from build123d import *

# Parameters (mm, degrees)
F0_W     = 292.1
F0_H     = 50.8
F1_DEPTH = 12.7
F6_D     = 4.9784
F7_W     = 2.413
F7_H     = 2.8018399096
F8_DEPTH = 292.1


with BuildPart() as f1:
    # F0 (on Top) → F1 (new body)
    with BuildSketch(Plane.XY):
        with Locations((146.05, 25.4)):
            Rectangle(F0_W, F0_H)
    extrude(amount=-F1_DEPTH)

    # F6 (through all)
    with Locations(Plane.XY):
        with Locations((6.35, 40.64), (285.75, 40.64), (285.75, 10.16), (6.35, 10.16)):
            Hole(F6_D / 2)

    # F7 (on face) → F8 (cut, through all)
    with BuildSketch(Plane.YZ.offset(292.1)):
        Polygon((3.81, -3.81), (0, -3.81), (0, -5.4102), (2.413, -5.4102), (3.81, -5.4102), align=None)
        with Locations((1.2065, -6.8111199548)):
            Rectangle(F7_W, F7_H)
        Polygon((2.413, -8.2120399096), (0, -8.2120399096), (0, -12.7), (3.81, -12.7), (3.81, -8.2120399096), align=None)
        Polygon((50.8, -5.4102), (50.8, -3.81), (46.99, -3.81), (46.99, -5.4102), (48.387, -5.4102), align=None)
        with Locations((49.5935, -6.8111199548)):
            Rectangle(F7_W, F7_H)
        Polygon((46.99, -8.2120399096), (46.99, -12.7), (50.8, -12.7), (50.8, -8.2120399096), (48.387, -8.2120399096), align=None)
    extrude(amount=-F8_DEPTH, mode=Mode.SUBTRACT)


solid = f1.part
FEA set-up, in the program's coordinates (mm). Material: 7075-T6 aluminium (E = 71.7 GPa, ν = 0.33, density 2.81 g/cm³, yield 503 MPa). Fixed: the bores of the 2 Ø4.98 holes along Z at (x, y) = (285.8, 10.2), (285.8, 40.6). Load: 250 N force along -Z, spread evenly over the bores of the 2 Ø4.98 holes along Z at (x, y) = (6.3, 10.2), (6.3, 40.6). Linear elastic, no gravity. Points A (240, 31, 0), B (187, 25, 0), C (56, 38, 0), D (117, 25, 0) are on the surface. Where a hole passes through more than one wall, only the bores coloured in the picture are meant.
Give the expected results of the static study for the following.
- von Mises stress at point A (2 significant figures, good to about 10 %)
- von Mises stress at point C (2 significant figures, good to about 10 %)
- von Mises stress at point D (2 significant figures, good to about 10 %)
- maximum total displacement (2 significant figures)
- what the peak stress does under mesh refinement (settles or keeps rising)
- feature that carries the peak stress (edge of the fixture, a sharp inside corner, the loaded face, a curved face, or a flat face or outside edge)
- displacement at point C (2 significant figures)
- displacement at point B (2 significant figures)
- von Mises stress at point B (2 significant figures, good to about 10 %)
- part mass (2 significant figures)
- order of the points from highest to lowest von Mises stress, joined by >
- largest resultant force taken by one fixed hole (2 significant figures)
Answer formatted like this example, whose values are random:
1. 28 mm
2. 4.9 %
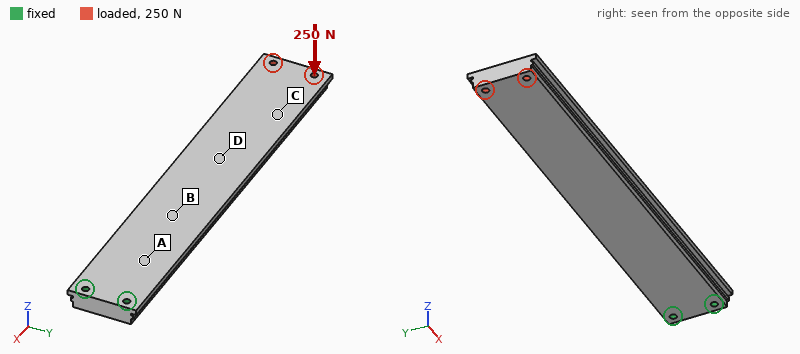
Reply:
1. 45 MPa
2. 9.6 MPa
3. 21 MPa
4. 3.4 mm
5. keeps rising
6. edge of the fixture
7. 2.4 mm
8. 0.57 mm
9. 35 MPa
10. 480 g
11. A > B > D > C
12. 210 N
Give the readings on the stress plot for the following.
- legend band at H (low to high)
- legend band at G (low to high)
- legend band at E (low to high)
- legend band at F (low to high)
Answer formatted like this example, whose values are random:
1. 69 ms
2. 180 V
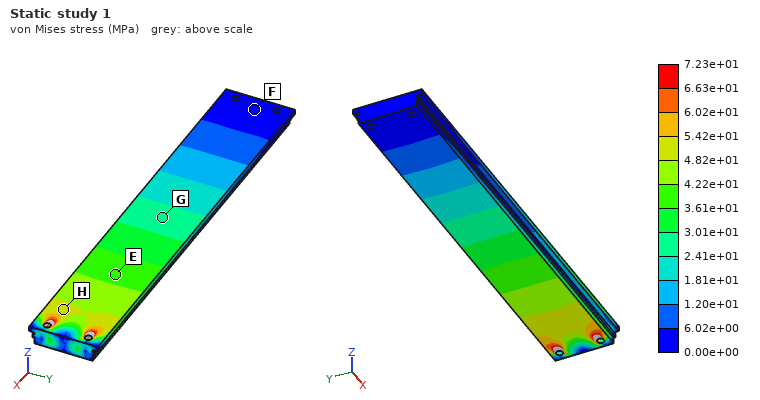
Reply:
1. 4.82e+01 to 5.42e+01 MPa
2. 2.41e+01 to 3.01e+01 MPa
3. 3.61e+01 to 4.22e+01 MPa
4. 0.00e+00 to 6.02e+00 MPa
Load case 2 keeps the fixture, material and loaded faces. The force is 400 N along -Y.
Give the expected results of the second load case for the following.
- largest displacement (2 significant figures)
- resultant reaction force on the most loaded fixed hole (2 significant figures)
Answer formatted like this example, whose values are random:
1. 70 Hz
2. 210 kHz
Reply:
1. 0.42 mm
2. 3.4 kN
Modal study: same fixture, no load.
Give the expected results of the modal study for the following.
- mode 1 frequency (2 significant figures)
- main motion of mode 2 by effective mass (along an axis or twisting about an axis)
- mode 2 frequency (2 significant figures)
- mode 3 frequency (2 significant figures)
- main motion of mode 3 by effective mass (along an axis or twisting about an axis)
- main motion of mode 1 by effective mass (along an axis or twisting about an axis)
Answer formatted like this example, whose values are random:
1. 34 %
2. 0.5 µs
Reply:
1. 130 Hz
2. along Y
3. 450 Hz
4. 780 Hz
5. along Z
6. along Z
